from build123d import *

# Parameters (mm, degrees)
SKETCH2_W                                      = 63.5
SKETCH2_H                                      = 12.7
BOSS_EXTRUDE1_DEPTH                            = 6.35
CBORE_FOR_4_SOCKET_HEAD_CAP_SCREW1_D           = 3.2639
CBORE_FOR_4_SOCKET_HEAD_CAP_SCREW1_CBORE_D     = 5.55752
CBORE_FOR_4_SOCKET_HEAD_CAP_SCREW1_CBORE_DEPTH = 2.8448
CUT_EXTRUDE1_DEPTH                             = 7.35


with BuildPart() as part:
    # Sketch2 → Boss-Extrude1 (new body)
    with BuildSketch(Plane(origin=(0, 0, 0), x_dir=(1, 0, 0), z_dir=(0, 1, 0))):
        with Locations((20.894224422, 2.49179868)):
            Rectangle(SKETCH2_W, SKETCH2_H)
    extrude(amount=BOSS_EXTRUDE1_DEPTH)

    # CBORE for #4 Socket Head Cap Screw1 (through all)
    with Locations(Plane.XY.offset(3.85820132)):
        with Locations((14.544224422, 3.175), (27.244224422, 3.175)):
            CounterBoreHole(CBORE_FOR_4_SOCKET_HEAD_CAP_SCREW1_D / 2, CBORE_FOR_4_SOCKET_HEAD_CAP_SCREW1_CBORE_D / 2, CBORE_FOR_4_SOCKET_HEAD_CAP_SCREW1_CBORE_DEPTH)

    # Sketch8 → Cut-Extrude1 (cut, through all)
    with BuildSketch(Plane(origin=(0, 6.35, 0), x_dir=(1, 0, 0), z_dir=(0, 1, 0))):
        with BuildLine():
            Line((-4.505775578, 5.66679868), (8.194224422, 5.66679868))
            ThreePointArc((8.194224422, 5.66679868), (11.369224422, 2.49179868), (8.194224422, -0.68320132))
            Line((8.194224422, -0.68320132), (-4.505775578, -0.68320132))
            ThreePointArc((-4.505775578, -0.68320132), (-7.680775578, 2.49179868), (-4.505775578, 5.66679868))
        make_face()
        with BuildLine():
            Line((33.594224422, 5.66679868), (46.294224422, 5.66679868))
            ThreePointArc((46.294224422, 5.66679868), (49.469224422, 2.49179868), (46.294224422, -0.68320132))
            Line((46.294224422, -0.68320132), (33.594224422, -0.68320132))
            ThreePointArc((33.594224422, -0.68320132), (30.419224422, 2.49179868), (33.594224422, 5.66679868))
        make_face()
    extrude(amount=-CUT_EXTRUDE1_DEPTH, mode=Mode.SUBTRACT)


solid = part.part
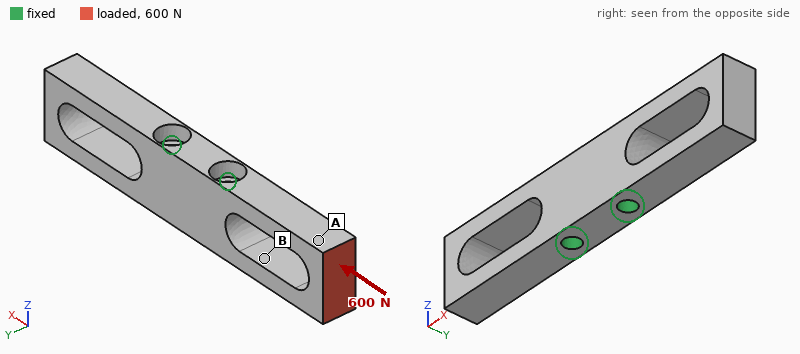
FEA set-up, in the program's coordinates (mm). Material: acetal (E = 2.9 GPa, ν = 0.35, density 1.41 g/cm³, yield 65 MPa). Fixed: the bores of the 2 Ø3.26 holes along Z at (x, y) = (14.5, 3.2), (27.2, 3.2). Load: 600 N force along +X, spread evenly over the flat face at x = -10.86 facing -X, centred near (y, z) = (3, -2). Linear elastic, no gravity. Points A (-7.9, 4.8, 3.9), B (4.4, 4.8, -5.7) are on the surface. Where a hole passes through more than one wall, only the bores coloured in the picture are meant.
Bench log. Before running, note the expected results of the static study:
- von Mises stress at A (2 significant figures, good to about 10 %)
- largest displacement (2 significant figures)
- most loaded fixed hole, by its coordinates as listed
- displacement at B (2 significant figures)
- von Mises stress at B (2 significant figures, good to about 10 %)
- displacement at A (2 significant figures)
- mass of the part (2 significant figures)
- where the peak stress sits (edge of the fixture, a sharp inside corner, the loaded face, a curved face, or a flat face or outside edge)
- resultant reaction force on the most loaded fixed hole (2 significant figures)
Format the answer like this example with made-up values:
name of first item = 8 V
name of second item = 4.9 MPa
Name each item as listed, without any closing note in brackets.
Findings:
von Mises stress at A = 9.7 MPa
largest displacement = 0.29 mm
most loaded fixed hole, by its coordinates as listed = (14.5, 3.2)
displacement at B = 0.050 mm
von Mises stress at B = 22 MPa
displacement at A = 0.25 mm
mass of the part = 4.8 g
where the peak stress sits = a curved face
resultant reaction force on the most loaded fixed hole = 550 N
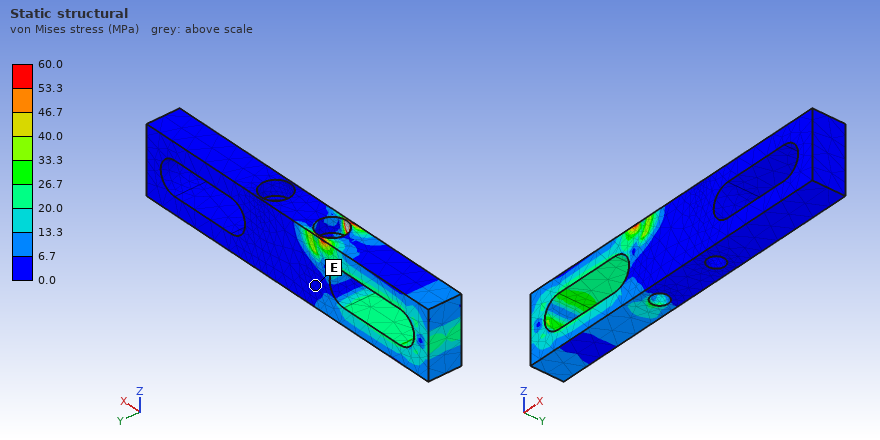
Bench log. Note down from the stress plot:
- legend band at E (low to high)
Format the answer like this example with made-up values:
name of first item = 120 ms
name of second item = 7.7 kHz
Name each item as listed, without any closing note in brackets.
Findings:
legend band at E = 0.0 to 6.7 MPa
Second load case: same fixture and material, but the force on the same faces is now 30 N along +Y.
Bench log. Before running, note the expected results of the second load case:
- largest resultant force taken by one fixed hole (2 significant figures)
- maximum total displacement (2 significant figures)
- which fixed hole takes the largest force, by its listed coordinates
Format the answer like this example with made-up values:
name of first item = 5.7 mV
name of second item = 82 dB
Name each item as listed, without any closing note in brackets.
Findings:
largest resultant force taken by one fixed hole = 46 N
maximum total displacement = 0.44 mm
which fixed hole takes the largest force, by its listed coordinates = (14.5, 3.2)
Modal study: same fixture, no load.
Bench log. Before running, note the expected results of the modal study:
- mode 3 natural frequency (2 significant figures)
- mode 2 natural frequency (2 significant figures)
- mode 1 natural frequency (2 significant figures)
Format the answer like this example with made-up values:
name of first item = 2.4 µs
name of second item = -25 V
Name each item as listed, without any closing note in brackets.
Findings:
mode 3 natural frequency = 1900 Hz
mode 2 natural frequency = 1800 Hz
mode 1 natural frequency = 1800 Hz
